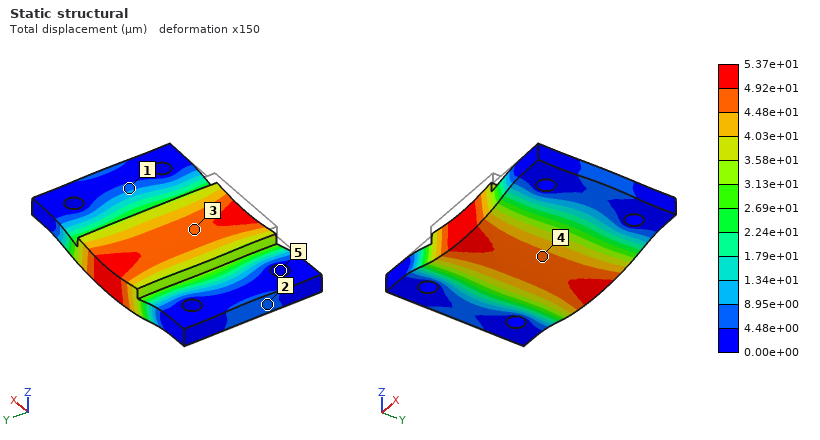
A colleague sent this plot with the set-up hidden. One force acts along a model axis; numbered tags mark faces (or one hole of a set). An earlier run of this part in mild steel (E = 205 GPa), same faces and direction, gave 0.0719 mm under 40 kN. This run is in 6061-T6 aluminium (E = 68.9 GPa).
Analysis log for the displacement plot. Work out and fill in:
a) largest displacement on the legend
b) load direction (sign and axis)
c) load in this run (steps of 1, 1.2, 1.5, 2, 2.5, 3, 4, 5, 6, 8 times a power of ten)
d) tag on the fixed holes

5.37e+01 µm
-Z
10 kN
5
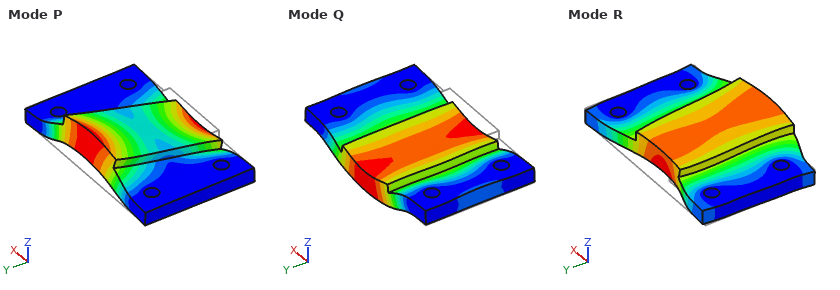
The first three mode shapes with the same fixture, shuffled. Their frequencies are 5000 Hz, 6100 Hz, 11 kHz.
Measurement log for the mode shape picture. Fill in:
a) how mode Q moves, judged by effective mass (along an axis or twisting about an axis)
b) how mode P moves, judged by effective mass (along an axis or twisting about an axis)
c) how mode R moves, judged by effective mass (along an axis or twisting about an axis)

along Z
twisting about X
along Y
